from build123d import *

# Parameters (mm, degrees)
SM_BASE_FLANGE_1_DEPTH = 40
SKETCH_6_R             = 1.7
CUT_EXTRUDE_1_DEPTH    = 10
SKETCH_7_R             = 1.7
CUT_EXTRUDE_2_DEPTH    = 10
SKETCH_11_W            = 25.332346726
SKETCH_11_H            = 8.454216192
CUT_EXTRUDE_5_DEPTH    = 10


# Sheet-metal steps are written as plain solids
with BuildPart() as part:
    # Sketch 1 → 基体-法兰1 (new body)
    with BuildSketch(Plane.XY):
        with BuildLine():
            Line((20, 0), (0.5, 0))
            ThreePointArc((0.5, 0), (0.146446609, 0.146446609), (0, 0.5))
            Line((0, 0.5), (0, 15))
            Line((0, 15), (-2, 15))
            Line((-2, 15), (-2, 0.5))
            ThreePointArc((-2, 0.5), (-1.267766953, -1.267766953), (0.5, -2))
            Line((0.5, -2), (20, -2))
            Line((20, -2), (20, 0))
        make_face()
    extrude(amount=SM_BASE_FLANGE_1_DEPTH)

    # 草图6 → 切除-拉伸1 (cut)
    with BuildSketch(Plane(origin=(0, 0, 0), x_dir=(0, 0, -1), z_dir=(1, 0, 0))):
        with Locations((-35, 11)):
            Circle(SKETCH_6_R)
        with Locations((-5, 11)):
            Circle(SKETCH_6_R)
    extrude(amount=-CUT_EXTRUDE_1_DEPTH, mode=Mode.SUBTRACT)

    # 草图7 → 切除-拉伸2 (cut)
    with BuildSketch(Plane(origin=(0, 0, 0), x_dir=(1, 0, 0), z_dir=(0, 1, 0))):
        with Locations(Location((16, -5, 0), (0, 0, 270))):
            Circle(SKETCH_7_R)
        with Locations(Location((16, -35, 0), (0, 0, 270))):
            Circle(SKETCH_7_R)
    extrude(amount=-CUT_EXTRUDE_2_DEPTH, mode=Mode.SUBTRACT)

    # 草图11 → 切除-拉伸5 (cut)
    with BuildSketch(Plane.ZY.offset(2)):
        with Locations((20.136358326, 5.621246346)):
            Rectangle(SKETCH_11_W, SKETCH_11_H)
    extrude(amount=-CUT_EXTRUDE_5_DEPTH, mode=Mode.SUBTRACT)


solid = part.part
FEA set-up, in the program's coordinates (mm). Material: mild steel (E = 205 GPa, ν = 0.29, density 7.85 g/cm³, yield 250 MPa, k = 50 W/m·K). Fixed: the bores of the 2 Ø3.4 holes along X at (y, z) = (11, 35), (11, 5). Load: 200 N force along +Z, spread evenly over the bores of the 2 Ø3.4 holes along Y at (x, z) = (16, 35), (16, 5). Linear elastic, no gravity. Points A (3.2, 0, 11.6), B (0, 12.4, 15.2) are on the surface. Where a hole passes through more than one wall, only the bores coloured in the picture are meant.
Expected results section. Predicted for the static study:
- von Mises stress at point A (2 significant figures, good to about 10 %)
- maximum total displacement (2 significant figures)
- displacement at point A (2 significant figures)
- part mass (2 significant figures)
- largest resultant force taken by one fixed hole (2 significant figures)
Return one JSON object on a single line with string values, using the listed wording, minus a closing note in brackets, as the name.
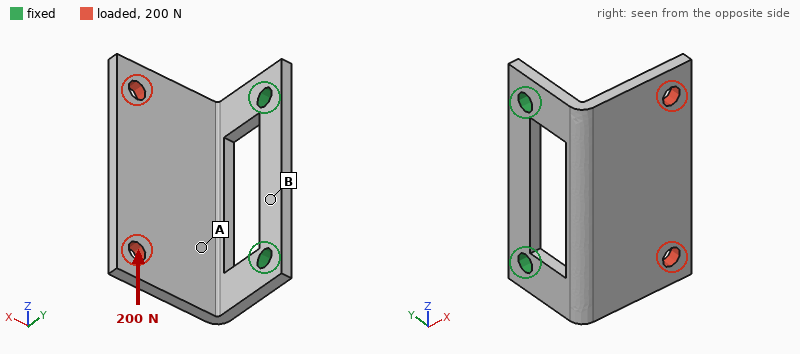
{"von Mises stress at point A": "30 MPa", "maximum total displacement": "50 µm", "displacement at point A": "15 µm", "part mass": "19 g", "largest resultant force taken by one fixed hole": "140 N"}
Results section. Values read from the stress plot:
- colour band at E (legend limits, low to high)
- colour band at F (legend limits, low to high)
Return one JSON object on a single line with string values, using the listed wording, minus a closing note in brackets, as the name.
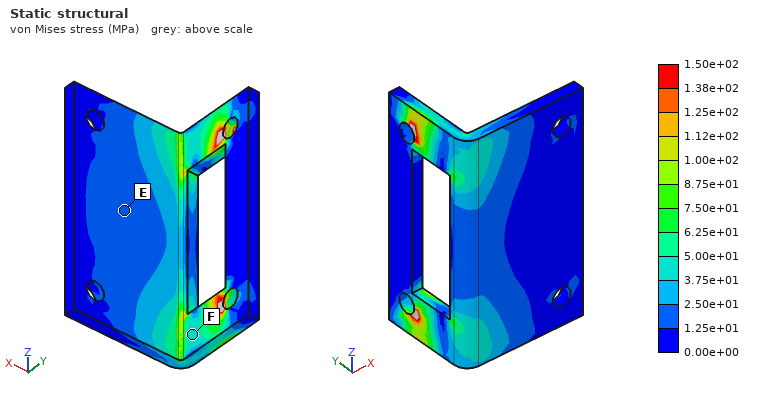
{"colour band at E": "1.25e+01 to 2.50e+01 MPa", "colour band at F": "3.75e+01 to 5.00e+01 MPa"}
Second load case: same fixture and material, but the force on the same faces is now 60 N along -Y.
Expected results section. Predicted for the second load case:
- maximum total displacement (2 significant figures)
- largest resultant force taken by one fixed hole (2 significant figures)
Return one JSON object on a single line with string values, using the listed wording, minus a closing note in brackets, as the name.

{"maximum total displacement": "0.15 mm", "largest resultant force taken by one fixed hole": "30 N"}
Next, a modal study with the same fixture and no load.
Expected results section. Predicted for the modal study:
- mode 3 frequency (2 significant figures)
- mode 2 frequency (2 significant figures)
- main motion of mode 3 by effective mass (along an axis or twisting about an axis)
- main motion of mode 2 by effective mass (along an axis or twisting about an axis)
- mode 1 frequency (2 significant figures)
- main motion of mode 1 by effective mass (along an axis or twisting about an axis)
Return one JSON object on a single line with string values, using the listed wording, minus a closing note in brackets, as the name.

{"mode 3 frequency": "4800 Hz", "mode 2 frequency": "3500 Hz", "main motion of mode 3 by effective mass": "along X", "main motion of mode 2 by effective mass": "along Z", "mode 1 frequency": "1300 Hz", "main motion of mode 1 by effective mass": "along Y"}
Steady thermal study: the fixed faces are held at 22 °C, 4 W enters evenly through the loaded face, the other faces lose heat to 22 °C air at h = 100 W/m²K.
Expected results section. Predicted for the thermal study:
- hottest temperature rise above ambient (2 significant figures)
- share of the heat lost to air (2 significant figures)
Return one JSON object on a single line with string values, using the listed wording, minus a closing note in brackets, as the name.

{"hottest temperature rise above ambient": "25 K", "share of the heat lost to air": "73 %"}
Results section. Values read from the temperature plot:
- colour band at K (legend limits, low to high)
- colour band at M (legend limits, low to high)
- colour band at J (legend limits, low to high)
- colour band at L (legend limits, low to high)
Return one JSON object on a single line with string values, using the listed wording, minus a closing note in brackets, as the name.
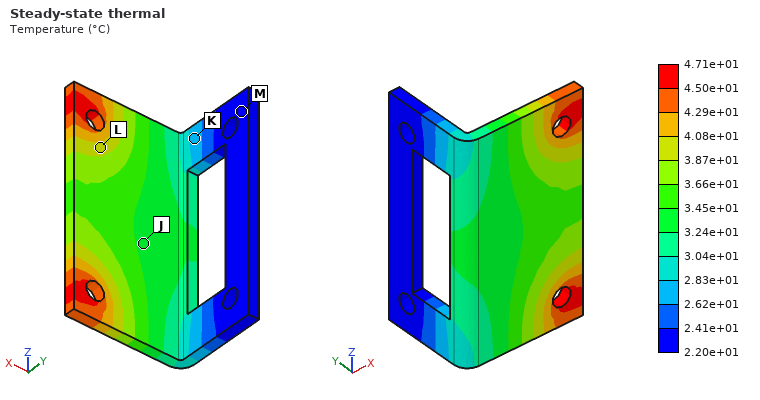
{"colour band at K": "2.62e+01 to 2.83e+01 °C", "colour band at M": "2.20e+01 to 2.41e+01 °C", "colour band at J": "3.24e+01 to 3.45e+01 °C", "colour band at L": "3.87e+01 to 4.08e+01 °C"}
